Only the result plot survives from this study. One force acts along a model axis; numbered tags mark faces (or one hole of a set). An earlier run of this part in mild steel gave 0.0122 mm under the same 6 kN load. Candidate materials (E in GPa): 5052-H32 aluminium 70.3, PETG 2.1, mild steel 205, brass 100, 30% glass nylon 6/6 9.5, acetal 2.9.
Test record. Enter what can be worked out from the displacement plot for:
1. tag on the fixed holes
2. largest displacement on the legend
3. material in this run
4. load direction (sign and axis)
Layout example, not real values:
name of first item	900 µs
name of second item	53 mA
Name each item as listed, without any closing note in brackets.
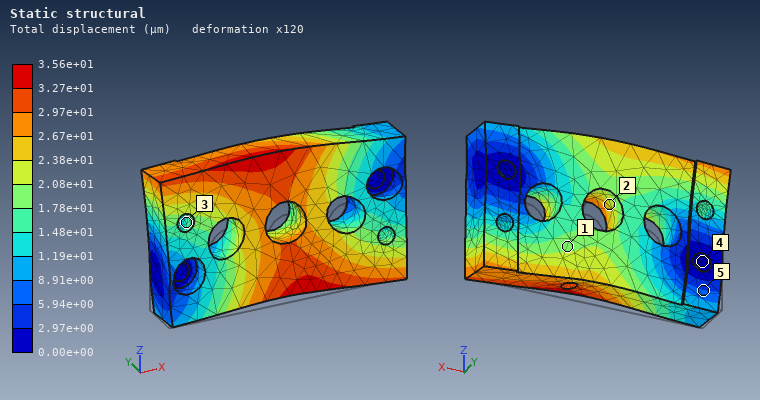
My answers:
tag on the fixed holes	4
largest displacement on the legend	3.56e+01 µm
material in this run	5052-H32 aluminium
load direction	+Z
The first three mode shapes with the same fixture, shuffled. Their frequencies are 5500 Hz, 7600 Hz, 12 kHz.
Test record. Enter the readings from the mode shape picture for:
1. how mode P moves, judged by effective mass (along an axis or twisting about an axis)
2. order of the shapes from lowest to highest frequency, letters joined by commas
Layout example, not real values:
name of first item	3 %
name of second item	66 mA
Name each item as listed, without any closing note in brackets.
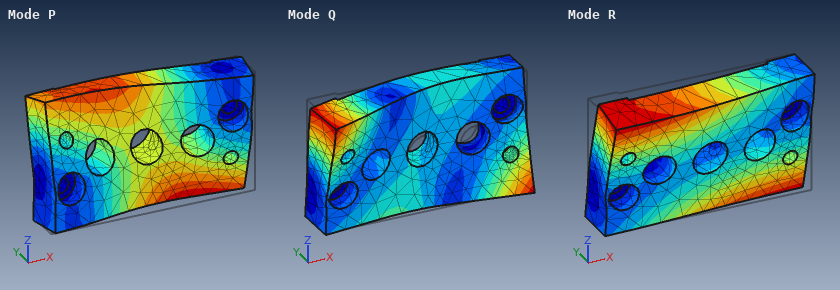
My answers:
how mode P moves, judged by effective mass	along Y
order of the shapes from lowest to highest frequency, letters joined by commas	R, P, Q
